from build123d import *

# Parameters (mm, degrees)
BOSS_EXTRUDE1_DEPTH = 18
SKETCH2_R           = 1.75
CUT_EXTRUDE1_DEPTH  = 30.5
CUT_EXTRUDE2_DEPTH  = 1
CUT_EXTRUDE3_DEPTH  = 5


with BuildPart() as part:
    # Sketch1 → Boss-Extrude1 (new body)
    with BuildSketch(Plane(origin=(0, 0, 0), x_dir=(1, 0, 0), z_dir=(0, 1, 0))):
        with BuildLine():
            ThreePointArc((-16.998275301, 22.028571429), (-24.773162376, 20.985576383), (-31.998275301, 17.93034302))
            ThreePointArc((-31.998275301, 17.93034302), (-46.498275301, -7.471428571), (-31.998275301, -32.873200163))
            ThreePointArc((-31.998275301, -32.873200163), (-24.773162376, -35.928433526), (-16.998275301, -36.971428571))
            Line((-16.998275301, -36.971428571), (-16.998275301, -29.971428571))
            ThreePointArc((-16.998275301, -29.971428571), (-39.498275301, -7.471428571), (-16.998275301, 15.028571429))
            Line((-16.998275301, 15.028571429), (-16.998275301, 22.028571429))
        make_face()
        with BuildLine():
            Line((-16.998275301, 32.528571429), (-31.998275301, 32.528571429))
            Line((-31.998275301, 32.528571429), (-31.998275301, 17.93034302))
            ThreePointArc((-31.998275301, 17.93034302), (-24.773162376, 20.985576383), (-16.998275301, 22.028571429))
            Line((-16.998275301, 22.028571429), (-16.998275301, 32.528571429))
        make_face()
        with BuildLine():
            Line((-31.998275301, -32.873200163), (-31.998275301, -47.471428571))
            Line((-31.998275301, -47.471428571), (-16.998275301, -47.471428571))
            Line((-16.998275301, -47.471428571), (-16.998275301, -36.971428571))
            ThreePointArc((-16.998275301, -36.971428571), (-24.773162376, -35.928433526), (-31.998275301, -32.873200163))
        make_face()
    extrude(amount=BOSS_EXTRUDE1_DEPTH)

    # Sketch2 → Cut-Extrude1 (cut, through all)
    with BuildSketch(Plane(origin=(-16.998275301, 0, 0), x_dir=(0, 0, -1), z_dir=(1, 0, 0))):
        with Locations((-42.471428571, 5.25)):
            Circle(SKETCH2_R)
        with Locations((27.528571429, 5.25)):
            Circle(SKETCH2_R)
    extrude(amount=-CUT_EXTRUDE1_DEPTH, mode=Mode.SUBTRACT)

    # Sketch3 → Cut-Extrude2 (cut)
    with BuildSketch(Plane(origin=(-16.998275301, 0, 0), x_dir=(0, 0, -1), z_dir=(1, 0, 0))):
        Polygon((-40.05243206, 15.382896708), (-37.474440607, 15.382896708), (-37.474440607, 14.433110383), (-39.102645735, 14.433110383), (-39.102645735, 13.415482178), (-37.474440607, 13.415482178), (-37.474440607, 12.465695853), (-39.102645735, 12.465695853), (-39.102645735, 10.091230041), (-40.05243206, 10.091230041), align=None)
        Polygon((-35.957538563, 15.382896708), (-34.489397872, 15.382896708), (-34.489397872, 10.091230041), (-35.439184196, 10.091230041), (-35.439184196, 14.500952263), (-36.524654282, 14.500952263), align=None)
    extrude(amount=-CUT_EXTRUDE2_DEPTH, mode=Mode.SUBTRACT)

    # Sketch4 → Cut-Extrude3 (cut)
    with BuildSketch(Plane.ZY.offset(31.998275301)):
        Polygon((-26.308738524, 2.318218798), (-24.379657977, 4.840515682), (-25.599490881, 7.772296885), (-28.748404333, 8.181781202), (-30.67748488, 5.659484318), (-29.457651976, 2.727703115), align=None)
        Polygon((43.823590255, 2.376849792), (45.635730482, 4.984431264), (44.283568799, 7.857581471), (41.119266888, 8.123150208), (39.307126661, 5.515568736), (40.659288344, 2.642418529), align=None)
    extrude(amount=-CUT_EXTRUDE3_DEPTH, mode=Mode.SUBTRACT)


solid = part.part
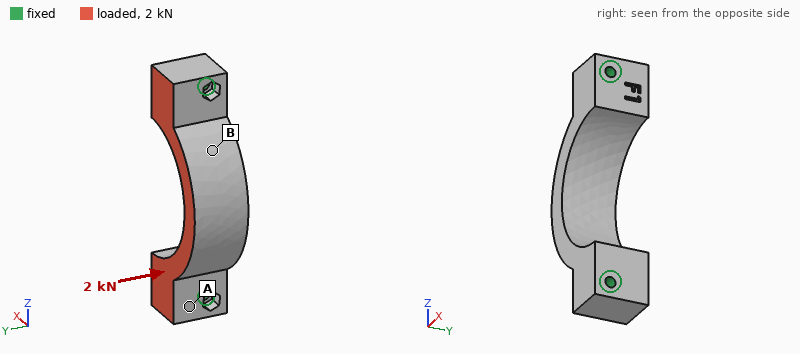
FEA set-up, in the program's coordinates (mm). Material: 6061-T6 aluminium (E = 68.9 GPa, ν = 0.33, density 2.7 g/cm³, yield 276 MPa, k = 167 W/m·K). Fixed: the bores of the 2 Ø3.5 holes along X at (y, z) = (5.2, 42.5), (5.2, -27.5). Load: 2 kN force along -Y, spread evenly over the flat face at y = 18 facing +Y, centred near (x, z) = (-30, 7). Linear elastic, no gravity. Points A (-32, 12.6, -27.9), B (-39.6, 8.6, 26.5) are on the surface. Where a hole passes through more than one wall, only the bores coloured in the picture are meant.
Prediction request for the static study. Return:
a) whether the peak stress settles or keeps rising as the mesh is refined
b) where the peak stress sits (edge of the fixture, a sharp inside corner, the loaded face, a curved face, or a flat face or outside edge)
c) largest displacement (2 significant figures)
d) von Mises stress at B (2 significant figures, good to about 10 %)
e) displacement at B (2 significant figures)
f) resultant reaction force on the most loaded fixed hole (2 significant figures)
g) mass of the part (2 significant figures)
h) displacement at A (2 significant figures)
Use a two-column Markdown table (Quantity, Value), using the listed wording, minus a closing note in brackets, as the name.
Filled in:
| Quantity | Value |
|---|---|
| whether the peak stress settles or keeps rising as the mesh is refined | keeps rising |
| where the peak stress sits | edge of the fixture |
| largest displacement | 47 µm |
| von Mises stress at B | 19 MPa |
| displacement at B | 28 µm |
| resultant reaction force on the most loaded fixed hole | 1.0 kN |
| mass of the part | 44 g |
| displacement at A | 7.2 µm |
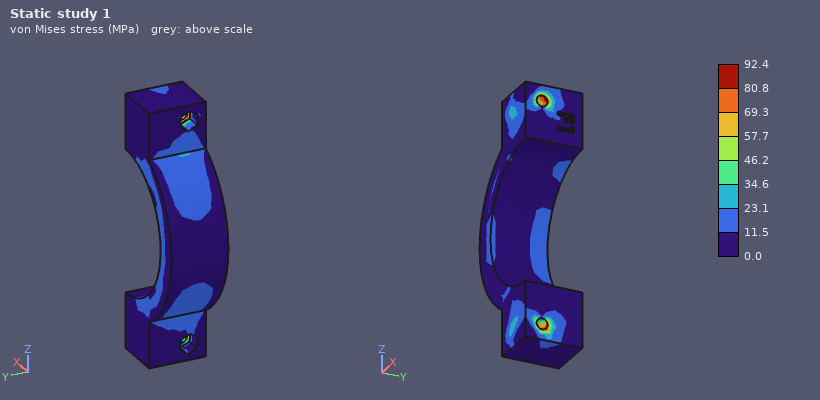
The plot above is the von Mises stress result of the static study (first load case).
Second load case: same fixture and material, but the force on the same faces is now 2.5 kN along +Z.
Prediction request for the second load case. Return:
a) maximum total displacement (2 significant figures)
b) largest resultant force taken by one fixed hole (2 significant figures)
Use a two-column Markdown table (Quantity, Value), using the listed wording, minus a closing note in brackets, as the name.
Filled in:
| Quantity | Value |
|---|---|
| maximum total displacement | 15 µm |
| largest resultant force taken by one fixed hole | 1.3 kN |
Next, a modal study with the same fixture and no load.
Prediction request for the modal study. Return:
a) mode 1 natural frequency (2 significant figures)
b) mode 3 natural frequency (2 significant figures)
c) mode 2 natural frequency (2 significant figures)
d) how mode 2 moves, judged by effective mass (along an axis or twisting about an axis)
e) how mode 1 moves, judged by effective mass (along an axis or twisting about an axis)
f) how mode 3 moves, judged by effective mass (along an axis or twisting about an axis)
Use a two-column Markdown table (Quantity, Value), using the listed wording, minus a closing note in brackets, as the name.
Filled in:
| Quantity | Value |
|---|---|
| mode 1 natural frequency | 6100 Hz |
| mode 3 natural frequency | 16 kHz |
| mode 2 natural frequency | 13 kHz |
| how mode 2 moves, judged by effective mass | along Z |
| how mode 1 moves, judged by effective mass | along Y |
| how mode 3 moves, judged by effective mass | along X |
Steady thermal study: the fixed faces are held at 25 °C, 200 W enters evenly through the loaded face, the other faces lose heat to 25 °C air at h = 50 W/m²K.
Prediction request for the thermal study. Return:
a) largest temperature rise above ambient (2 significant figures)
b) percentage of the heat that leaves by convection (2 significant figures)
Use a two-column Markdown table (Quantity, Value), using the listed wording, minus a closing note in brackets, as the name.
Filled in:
| Quantity | Value |
|---|---|
| largest temperature rise above ambient | 66 K |
| percentage of the heat that leaves by convection | 4.2 % |
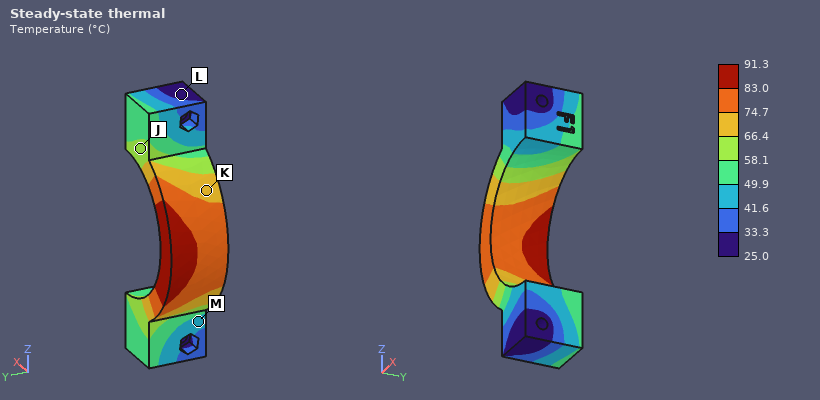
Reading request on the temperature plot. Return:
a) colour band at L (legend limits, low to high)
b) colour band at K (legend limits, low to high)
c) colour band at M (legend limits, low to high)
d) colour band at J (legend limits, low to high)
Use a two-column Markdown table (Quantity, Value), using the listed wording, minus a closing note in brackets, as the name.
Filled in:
| Quantity | Value |
|---|---|
| colour band at L | 25.0 to 33.3 °C |
| colour band at K | 66.4 to 74.7 °C |
| colour band at M | 41.6 to 49.9 °C |
| colour band at J | 58.1 to 66.4 °C |
